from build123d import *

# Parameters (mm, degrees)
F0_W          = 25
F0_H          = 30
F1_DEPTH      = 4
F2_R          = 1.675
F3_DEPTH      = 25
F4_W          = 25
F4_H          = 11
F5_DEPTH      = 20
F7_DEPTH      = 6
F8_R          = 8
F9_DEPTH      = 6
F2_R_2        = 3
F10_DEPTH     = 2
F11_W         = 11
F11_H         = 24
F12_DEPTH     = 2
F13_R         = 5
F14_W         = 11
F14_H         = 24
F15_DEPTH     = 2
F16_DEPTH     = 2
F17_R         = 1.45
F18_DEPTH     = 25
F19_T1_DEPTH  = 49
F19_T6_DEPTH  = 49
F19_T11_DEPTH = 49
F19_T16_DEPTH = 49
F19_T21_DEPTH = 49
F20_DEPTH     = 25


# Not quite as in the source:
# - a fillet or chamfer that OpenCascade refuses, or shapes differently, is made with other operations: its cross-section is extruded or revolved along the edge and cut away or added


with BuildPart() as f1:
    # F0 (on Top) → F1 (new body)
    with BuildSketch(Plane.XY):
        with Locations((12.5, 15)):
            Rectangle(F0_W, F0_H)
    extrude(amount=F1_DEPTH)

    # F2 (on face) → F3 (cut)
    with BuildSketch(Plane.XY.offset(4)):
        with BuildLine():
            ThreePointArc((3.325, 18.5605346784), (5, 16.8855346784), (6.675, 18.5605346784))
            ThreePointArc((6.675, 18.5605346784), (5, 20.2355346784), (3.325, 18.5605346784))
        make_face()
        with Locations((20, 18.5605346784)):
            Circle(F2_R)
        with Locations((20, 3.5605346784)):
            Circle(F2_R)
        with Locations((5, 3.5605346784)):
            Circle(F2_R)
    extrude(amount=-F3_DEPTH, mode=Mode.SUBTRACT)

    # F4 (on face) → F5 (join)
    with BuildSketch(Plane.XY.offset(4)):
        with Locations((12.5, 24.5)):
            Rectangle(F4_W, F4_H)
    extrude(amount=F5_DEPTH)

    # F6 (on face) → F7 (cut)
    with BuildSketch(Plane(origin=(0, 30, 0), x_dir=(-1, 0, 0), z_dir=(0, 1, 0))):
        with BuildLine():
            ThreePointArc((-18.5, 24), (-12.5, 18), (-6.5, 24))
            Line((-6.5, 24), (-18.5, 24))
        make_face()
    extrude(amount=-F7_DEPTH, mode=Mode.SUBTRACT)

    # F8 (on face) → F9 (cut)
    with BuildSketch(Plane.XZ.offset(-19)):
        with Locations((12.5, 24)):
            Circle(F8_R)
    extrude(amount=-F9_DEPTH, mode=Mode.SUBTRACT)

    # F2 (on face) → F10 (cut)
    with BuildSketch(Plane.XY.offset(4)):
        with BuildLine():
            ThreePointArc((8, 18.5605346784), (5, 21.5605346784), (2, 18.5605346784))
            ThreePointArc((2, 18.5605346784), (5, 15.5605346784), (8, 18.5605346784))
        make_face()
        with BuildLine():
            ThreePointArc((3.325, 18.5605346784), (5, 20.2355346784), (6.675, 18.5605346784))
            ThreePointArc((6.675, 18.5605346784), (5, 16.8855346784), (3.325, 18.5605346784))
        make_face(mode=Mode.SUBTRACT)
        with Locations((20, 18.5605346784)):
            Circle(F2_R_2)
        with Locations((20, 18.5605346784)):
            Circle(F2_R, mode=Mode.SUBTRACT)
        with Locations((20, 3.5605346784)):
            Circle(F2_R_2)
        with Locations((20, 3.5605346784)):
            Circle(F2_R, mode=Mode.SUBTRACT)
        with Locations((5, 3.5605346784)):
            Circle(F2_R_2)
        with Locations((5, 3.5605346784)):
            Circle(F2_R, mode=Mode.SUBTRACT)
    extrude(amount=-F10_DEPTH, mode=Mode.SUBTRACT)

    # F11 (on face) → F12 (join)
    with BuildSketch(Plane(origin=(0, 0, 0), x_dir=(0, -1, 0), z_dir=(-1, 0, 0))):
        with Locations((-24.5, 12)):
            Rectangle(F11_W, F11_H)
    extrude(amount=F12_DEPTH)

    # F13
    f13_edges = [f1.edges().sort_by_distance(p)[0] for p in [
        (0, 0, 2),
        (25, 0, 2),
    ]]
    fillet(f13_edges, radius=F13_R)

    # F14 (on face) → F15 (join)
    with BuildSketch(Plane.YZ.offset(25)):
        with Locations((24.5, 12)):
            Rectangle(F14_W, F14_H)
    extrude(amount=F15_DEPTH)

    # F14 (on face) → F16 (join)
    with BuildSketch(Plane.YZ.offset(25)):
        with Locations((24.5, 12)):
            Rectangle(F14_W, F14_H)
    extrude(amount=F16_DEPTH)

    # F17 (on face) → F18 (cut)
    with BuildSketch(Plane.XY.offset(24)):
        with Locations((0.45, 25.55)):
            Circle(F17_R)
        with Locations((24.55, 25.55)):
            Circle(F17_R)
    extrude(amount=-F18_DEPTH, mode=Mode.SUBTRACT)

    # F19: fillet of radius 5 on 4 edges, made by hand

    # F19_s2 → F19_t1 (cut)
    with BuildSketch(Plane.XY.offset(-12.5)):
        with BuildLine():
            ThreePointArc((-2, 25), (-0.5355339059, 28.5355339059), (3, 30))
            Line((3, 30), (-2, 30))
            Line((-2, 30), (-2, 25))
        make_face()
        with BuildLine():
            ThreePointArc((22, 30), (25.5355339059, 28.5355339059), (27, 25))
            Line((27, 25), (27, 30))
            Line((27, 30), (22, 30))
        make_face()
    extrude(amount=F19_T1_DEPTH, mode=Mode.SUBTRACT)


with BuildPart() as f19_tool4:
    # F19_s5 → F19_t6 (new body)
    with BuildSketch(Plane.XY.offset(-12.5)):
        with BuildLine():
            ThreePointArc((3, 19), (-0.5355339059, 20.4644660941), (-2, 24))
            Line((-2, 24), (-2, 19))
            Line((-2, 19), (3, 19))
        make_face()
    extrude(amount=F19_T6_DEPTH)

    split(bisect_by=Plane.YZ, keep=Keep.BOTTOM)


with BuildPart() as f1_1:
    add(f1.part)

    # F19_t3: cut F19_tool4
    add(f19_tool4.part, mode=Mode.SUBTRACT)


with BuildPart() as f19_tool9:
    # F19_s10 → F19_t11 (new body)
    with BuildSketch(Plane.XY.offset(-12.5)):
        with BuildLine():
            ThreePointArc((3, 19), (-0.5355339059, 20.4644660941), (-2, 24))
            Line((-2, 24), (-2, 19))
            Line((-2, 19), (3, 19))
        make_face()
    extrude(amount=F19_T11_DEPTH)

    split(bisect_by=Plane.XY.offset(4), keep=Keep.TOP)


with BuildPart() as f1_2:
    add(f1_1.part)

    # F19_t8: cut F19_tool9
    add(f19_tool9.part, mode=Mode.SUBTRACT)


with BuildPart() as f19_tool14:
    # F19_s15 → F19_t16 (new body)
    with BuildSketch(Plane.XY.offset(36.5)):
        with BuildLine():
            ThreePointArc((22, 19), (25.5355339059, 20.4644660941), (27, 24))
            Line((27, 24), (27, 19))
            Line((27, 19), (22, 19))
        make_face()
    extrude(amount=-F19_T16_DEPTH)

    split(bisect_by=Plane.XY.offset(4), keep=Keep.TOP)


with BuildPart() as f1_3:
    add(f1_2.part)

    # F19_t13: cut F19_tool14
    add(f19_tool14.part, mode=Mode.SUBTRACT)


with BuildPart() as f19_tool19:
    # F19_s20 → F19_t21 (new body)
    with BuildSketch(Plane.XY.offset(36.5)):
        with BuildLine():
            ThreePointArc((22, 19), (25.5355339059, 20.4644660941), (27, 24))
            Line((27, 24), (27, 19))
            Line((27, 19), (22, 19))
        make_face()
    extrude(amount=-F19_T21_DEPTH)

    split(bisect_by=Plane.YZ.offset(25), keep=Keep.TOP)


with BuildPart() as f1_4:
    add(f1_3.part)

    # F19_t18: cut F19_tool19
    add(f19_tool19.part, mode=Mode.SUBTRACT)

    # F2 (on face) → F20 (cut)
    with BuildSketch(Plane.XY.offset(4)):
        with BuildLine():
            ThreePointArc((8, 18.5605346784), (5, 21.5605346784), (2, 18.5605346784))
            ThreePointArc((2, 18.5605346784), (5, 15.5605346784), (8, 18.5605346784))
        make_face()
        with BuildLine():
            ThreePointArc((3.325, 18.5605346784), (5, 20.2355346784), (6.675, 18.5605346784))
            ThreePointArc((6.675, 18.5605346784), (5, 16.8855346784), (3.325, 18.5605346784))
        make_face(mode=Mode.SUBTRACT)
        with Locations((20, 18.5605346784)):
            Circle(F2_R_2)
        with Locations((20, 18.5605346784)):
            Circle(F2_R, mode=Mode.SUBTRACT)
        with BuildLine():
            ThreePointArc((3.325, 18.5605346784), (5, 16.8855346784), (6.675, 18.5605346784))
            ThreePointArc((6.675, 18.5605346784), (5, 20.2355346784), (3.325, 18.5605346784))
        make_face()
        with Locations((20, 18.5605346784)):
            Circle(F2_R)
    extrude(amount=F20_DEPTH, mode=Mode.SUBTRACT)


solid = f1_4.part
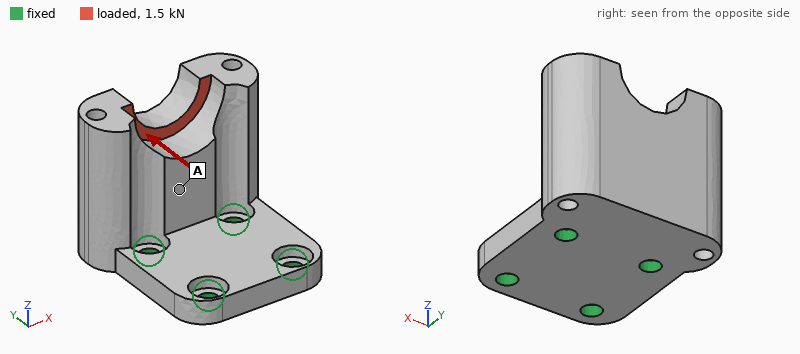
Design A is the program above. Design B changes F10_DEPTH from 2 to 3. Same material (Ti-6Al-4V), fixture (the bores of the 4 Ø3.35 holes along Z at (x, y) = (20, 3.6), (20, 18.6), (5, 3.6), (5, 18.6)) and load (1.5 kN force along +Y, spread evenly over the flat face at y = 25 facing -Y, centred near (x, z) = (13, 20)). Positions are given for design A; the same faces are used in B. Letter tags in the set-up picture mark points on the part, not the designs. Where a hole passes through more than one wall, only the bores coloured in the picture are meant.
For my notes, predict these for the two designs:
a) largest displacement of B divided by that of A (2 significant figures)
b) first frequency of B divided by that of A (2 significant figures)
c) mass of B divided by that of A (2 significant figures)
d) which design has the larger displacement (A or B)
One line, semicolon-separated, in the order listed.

1.2; 0.88; 0.99; B
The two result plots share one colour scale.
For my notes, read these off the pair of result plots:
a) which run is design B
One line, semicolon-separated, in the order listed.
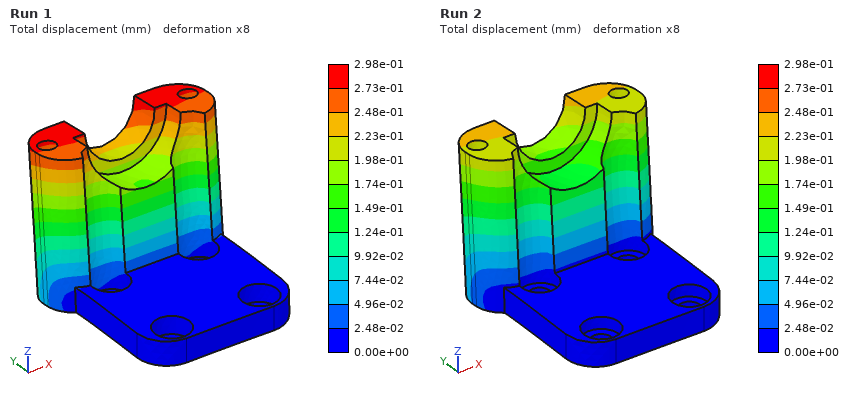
Run 1
